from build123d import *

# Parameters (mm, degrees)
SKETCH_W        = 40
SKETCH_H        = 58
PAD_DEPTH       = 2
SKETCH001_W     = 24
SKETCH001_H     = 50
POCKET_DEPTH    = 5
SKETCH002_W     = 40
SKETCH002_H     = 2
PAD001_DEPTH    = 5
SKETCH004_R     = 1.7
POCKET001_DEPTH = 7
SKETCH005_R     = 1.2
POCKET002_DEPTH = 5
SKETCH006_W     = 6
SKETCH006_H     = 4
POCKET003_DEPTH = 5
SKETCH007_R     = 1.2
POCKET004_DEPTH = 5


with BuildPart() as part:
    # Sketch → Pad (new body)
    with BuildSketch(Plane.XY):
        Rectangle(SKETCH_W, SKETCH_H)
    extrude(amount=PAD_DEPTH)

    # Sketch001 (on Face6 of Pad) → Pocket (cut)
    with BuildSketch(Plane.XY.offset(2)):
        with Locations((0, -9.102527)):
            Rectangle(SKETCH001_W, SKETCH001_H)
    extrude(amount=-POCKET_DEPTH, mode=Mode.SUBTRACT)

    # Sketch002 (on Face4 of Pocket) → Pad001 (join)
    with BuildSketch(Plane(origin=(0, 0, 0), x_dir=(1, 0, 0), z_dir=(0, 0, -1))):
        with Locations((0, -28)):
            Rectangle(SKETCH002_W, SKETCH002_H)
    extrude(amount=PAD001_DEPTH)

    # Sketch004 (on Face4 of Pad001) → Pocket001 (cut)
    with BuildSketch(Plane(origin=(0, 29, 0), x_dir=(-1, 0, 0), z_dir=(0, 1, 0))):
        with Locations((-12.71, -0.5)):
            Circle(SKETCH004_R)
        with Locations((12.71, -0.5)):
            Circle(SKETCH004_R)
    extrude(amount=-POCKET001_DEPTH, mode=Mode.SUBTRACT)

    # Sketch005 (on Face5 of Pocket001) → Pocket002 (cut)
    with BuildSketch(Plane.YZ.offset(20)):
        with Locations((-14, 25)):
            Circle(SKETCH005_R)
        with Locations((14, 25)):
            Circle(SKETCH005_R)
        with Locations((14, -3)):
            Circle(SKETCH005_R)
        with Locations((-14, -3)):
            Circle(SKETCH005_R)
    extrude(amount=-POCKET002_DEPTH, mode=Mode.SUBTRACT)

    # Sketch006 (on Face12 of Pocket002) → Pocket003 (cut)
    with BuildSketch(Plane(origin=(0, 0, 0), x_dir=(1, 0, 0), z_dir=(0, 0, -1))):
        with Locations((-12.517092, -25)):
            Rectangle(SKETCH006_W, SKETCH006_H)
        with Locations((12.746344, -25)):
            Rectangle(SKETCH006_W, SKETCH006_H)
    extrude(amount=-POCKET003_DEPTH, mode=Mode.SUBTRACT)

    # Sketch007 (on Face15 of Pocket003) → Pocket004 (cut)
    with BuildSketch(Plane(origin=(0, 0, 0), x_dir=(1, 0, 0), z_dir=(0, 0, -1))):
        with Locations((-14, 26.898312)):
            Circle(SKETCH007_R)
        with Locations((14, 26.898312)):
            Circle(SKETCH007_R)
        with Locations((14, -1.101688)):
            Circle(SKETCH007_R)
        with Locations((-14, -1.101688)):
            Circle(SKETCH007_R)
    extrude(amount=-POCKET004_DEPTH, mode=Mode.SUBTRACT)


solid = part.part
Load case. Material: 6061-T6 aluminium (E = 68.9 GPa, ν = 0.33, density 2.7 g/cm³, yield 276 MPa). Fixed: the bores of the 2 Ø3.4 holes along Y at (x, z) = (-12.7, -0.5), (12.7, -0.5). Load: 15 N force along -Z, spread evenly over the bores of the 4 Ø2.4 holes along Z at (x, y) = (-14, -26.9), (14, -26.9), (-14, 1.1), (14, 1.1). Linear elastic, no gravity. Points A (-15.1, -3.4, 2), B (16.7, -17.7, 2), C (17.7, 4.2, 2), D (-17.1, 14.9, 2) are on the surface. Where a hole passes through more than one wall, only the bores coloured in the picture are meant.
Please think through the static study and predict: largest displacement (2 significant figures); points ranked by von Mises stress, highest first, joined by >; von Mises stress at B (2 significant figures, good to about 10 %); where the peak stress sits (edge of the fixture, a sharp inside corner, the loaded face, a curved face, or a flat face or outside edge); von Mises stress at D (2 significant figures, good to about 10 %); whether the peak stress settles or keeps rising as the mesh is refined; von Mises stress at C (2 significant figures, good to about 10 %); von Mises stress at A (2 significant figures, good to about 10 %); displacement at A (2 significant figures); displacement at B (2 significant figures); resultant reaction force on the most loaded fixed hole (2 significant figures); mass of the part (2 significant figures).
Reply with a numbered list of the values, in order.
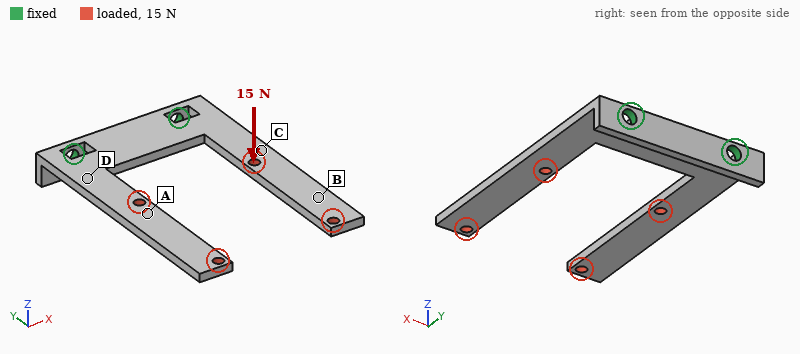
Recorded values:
1. 0.74 mm
2. D > C > A > B
3. 6.6 MPa
4. a sharp inside corner
5. 36 MPa
6. keeps rising
7. 26 MPa
8. 16 MPa
9. 0.28 mm
10. 0.53 mm
11. 9.1 N
12. 7.3 g
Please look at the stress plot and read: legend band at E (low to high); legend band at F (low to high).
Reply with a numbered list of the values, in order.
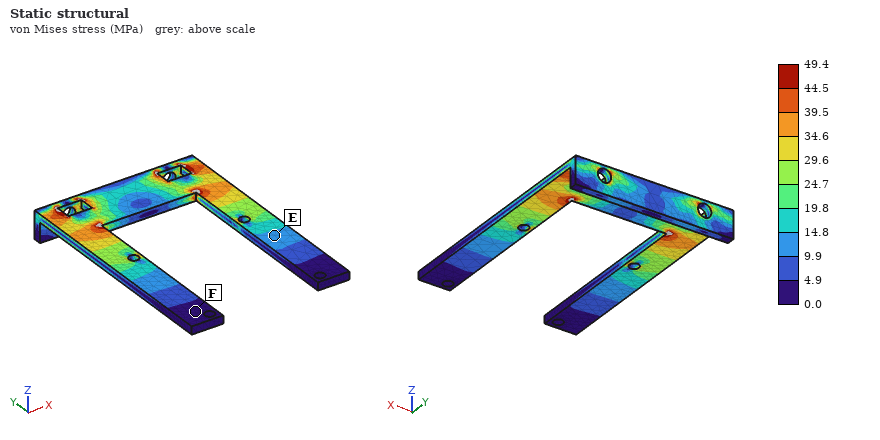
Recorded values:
1. 9.9 to 14.8 MPa
2. 0.0 to 4.9 MPa
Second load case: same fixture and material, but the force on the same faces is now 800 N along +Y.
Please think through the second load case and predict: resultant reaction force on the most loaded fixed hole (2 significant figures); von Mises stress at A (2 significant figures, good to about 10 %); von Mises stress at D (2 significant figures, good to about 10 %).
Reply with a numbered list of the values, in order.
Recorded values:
1. 400 N
2. 14 MPa
3. 14 MPa
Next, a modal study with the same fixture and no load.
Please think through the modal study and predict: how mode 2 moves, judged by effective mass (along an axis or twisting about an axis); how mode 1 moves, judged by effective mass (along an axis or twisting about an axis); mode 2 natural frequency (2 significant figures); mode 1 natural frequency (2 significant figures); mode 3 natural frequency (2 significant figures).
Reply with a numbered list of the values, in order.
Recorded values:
1. twisting about Y
2. along Z
3. 560 Hz
4. 530 Hz
5. 2500 Hz
